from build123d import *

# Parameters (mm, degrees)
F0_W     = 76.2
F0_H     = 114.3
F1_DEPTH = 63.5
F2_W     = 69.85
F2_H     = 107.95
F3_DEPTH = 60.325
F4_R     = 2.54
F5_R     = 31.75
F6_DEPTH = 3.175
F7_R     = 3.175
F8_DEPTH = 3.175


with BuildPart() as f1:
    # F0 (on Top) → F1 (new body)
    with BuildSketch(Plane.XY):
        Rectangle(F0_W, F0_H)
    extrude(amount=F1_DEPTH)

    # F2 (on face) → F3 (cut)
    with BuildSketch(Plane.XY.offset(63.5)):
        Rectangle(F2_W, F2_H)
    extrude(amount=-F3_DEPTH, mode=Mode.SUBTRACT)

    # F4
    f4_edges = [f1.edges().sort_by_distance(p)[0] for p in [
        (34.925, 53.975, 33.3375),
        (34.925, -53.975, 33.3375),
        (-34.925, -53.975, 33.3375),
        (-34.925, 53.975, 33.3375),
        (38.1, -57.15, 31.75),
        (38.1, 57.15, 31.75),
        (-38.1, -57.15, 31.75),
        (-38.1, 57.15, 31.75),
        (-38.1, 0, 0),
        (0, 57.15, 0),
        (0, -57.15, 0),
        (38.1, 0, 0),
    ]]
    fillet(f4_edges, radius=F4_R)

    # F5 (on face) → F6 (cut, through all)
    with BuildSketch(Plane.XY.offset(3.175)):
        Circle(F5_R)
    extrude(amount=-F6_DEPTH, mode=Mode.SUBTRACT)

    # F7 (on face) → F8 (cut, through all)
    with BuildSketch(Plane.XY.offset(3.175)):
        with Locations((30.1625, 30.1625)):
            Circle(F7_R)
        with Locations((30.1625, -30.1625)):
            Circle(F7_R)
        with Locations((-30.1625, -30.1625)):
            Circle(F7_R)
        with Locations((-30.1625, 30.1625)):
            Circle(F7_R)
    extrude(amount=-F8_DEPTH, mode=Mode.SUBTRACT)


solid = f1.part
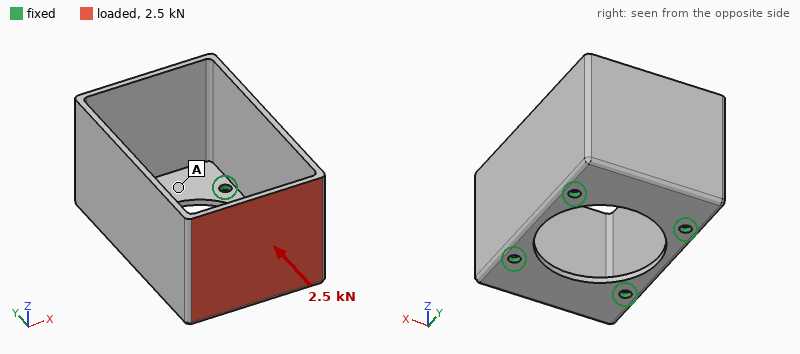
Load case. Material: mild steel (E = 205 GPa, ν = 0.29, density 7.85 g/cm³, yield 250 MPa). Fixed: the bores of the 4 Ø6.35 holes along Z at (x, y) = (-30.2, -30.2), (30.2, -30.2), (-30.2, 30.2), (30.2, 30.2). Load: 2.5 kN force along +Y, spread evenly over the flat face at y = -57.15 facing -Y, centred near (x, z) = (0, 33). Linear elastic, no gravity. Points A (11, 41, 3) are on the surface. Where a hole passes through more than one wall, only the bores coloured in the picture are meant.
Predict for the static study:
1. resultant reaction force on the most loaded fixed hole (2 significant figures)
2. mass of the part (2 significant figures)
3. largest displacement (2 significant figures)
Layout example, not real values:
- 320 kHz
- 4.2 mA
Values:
- 1.1 kN
- 680 g
- 0.17 mm
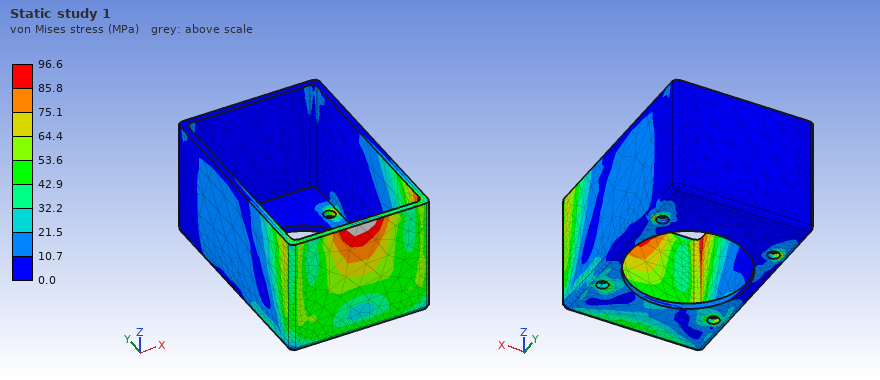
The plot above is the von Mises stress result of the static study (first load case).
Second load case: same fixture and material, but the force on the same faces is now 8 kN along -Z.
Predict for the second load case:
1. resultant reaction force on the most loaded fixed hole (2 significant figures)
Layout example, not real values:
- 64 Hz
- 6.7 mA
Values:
- 5.7 kN
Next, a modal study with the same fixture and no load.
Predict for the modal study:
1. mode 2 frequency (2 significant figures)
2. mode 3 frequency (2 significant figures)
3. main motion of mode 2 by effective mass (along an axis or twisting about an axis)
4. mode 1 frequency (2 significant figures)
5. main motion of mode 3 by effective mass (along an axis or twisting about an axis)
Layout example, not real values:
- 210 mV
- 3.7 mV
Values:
- 1400 Hz
- 2300 Hz
- along X
- 1300 Hz
- along Y
